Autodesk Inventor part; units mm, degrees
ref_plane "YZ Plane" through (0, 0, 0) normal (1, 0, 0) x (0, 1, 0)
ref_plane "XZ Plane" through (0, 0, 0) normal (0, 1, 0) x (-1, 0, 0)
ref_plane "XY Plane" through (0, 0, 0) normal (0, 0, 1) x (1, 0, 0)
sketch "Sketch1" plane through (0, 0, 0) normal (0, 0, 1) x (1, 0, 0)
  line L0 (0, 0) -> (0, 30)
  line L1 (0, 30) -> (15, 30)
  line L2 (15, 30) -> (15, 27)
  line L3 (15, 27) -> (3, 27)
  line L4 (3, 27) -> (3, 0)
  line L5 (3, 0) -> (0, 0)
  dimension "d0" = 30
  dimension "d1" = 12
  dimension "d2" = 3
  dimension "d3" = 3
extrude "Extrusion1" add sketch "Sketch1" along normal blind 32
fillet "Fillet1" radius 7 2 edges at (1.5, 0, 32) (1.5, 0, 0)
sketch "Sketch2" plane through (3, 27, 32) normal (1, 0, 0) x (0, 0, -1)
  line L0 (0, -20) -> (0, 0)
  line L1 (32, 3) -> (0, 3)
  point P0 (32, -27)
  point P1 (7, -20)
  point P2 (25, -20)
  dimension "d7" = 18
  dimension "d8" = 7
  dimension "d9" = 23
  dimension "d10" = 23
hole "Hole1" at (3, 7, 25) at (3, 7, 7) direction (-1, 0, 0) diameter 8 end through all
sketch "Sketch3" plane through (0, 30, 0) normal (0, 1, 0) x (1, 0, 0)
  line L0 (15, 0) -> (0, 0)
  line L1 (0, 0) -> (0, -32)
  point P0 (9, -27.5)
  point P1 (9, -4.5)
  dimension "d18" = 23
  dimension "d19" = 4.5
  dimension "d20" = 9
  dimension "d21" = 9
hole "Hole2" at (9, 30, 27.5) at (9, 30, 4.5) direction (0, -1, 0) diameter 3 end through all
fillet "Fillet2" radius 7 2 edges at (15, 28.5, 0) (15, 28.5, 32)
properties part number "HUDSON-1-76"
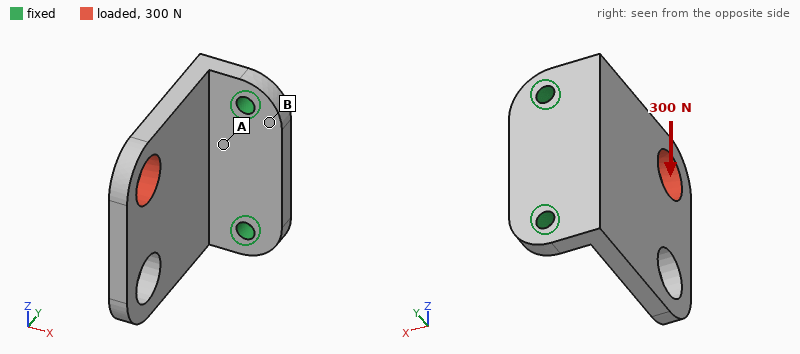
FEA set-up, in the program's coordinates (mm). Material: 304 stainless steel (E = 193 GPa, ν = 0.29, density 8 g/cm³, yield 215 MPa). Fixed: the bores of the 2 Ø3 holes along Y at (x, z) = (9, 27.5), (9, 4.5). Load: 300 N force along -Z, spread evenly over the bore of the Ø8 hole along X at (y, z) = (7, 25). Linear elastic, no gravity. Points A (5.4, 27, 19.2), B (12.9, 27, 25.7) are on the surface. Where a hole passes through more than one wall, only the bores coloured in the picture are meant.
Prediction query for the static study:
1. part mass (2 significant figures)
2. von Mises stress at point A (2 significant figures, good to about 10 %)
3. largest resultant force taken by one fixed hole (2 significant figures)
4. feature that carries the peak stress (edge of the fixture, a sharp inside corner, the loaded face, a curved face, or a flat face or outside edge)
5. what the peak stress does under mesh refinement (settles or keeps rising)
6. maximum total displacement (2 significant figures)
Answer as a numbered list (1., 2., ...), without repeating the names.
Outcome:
1. 28 g
2. 25 MPa
3. 320 N
4. edge of the fixture
5. keeps rising
6. 16 µm
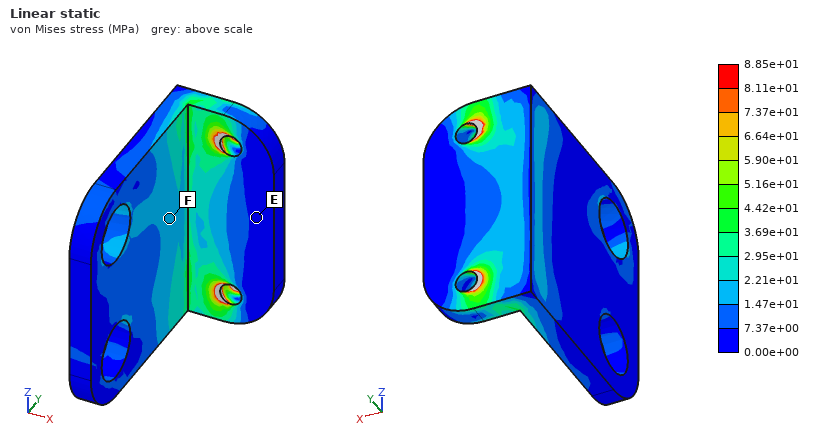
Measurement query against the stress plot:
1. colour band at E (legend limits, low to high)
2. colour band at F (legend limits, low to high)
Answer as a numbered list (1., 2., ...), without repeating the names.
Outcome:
1. 0.00e+00 to 7.37e+00 MPa
2. 1.47e+01 to 2.21e+01 MPa
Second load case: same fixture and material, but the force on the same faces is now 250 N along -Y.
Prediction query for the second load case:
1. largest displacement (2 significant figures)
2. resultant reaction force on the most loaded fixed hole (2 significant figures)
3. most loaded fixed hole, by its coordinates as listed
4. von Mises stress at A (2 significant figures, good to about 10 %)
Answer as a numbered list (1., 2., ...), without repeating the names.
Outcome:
1. 20 µm
2. 220 N
3. (9, 27.5)
4. 14 MPa
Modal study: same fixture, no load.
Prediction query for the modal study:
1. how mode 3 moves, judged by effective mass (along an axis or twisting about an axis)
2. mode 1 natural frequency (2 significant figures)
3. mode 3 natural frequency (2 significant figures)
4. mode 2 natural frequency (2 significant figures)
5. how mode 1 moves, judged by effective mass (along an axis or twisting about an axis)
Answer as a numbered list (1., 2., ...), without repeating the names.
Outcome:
1. along Z
2. 2400 Hz
3. 9000 Hz
4. 6200 Hz
5. along X
